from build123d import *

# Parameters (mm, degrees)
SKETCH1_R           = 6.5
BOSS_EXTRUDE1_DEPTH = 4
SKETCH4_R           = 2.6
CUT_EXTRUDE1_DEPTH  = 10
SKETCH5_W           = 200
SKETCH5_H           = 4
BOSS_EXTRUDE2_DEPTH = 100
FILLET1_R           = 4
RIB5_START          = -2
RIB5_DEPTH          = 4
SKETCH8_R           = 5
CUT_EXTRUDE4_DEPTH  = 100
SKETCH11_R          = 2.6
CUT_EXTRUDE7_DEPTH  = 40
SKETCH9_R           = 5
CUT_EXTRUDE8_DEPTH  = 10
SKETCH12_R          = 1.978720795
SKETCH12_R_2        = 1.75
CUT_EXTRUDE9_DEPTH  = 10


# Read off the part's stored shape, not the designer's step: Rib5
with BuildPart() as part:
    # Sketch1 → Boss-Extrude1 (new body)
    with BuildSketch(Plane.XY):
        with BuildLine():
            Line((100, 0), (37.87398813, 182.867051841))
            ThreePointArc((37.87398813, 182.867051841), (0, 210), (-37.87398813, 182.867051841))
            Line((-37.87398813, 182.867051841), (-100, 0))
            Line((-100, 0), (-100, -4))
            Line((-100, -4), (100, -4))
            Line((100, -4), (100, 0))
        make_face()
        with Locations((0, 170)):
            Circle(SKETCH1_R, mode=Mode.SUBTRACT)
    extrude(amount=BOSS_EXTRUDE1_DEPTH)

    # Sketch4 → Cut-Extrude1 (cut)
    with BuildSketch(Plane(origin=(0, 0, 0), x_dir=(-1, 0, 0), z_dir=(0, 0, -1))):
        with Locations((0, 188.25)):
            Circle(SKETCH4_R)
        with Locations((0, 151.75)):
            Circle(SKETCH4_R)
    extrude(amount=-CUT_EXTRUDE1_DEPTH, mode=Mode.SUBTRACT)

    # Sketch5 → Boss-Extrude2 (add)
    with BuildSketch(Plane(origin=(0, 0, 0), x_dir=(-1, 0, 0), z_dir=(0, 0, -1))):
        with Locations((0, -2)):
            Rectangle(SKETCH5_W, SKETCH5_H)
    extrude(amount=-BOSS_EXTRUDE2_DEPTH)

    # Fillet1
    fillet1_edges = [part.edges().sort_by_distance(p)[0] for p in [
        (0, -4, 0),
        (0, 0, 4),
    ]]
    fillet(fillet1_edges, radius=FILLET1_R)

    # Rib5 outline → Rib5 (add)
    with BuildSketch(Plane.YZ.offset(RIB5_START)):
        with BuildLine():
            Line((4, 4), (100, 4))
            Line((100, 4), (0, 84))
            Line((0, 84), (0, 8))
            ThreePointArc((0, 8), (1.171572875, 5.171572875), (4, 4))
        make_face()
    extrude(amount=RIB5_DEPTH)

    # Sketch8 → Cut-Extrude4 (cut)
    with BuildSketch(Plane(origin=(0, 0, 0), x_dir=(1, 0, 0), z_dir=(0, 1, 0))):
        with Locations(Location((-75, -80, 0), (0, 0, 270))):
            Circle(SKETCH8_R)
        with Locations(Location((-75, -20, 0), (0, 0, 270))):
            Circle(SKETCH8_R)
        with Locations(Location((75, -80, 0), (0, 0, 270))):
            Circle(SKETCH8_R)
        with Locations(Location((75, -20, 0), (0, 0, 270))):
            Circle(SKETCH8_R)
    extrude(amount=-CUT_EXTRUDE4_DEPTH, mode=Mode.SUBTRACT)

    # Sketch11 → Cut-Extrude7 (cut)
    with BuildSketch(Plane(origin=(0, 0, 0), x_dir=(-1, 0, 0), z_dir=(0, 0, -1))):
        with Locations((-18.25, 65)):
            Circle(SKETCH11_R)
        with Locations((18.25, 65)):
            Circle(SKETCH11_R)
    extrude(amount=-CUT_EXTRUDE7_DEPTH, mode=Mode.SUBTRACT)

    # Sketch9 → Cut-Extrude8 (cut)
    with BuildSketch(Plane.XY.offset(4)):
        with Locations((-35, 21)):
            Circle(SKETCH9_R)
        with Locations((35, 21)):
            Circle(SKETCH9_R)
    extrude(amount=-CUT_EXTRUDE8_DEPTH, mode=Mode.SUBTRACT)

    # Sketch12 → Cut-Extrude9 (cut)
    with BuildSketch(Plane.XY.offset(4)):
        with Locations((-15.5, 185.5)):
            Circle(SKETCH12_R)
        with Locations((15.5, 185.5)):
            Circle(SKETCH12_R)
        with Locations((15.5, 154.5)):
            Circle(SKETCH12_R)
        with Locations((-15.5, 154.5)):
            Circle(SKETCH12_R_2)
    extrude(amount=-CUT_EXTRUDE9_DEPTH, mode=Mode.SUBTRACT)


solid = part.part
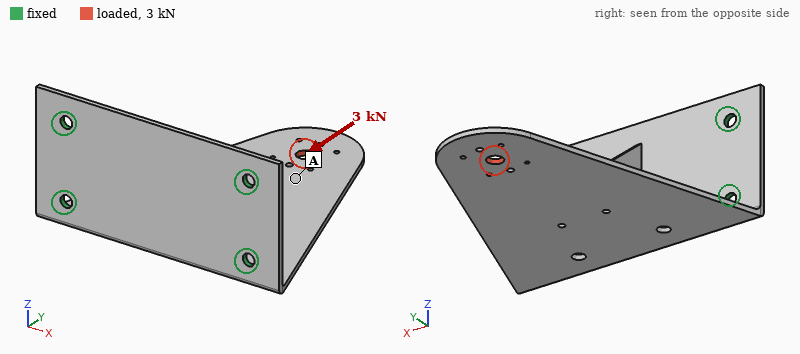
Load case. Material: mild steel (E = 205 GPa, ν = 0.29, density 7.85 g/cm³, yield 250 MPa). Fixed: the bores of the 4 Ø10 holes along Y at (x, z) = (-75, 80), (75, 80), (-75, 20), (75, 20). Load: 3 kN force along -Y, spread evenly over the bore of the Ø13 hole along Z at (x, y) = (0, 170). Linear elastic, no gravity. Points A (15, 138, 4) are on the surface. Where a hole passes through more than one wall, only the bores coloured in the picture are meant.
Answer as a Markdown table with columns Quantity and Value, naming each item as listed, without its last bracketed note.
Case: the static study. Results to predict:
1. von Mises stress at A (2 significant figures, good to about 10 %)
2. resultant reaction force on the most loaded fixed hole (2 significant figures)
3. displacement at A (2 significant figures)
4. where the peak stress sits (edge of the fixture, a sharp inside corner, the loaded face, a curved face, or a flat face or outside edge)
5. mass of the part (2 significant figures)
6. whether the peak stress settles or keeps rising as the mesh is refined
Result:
| Quantity | Value |
|---|---|
| von Mises stress at A | 11 MPa |
| resultant reaction force on the most loaded fixed hole | 1.7 kN |
| displacement at A | 0.12 mm |
| where the peak stress sits | edge of the fixture |
| mass of the part | 1.6 kg |
| whether the peak stress settles or keeps rising as the mesh is refined | keeps rising |
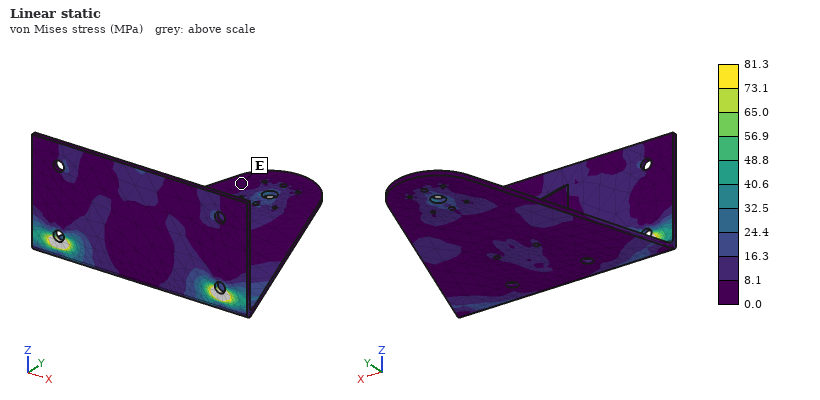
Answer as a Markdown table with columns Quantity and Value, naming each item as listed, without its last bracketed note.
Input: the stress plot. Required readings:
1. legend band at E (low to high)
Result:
| Quantity | Value |
|---|---|
| legend band at E | 0.0 to 8.1 MPa |
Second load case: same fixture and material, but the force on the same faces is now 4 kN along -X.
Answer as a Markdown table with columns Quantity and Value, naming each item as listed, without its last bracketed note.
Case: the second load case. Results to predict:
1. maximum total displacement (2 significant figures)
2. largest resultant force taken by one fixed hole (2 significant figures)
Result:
| Quantity | Value |
|---|---|
| maximum total displacement | 0.33 mm |
| largest resultant force taken by one fixed hole | 5.0 kN |
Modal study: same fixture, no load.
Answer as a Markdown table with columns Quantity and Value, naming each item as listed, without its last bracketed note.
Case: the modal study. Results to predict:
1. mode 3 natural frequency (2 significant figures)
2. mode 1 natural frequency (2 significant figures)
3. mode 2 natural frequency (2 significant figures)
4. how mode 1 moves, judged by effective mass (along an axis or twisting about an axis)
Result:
| Quantity | Value |
|---|---|
| mode 3 natural frequency | 560 Hz |
| mode 1 natural frequency | 200 Hz |
| mode 2 natural frequency | 440 Hz |
| how mode 1 moves, judged by effective mass | along Z |
